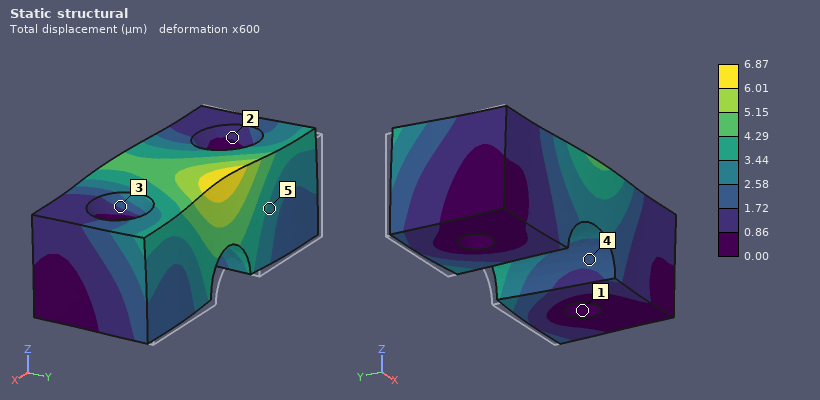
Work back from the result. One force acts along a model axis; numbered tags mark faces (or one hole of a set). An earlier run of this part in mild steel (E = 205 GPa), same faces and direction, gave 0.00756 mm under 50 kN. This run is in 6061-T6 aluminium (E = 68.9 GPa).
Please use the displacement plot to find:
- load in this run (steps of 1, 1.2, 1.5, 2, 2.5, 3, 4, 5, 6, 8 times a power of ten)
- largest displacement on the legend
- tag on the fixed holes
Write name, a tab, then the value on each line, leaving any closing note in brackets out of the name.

load in this run	15 kN
largest displacement on the legend	6.87 µm
tag on the fixed holes	1
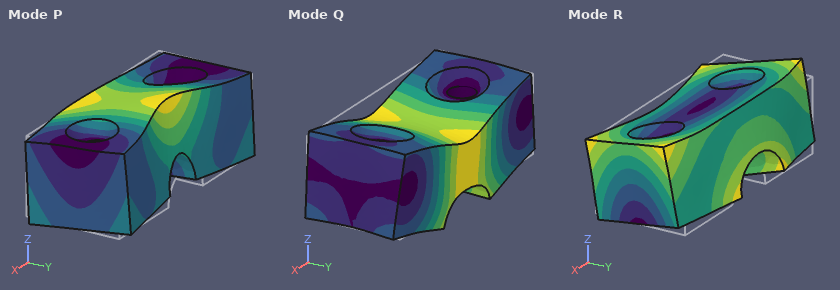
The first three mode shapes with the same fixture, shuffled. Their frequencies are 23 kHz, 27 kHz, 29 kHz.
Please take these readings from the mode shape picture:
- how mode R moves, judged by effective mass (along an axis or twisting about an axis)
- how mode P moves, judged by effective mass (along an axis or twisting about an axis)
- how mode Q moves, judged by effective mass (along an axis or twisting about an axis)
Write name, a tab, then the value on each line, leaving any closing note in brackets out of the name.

how mode R moves, judged by effective mass	twisting about X
how mode P moves, judged by effective mass	along Y
how mode Q moves, judged by effective mass	along Z
